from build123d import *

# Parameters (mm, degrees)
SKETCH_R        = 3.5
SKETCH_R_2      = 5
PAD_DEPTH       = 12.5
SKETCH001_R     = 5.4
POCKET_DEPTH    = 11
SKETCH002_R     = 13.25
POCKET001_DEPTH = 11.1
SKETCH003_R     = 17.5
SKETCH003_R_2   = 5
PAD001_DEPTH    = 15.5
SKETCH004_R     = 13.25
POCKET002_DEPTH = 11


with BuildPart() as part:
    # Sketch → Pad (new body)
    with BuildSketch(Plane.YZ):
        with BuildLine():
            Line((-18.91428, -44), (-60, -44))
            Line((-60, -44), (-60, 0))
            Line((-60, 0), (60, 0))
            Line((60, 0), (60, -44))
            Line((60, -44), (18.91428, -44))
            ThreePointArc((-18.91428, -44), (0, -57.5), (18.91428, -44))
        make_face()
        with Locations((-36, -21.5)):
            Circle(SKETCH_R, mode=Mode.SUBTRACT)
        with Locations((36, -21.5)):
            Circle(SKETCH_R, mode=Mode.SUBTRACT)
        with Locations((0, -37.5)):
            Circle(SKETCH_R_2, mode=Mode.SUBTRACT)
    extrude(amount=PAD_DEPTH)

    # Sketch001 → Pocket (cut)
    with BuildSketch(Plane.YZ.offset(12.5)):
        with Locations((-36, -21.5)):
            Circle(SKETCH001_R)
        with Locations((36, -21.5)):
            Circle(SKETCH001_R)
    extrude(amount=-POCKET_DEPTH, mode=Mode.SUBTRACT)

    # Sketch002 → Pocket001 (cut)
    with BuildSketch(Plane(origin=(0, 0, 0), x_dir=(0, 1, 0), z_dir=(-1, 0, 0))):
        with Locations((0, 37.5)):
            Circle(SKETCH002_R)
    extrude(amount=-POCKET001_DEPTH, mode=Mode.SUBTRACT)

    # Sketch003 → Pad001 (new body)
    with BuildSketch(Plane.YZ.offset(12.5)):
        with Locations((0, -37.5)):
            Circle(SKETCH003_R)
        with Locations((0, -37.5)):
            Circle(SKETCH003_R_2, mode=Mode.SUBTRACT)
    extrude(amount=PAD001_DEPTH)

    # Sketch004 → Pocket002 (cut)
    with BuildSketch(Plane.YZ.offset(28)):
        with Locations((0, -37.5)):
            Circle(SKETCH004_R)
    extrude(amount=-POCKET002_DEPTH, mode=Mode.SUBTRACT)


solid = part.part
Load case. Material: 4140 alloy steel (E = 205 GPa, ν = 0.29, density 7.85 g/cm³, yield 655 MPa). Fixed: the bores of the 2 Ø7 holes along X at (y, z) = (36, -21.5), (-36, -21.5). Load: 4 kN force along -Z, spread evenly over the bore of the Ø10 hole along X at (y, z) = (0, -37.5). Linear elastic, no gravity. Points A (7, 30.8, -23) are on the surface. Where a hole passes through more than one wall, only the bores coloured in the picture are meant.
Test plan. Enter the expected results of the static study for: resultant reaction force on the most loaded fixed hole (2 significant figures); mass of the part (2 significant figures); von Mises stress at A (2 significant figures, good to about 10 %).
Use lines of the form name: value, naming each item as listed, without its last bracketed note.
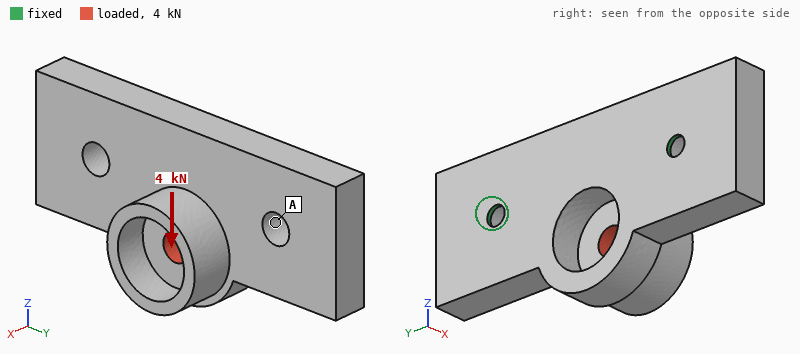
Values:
resultant reaction force on the most loaded fixed hole: 2.0 kN
mass of the part: 560 g
von Mises stress at A: 68 MPa
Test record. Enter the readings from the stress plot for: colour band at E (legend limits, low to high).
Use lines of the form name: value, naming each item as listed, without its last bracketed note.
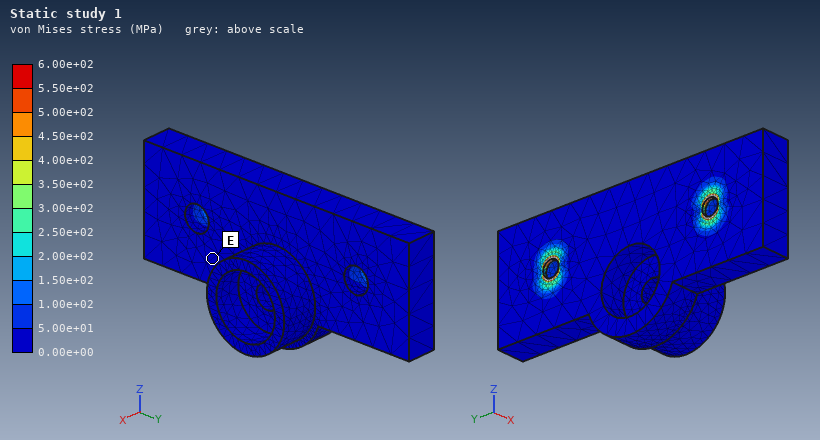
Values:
colour band at E: 0.00e+00 to 5.00e+01 MPa
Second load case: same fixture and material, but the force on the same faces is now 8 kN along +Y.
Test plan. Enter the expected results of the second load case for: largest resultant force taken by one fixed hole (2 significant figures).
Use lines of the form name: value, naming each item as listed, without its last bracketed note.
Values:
largest resultant force taken by one fixed hole: 4.6 kN
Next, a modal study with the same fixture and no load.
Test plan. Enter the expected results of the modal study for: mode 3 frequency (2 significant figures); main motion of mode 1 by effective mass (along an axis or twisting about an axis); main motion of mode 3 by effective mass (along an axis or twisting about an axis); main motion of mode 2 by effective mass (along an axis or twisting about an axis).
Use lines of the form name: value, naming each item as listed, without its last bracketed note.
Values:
mode 3 frequency: 5900 Hz
main motion of mode 1 by effective mass: along Z
main motion of mode 3 by effective mass: twisting about X
main motion of mode 2 by effective mass: along X
